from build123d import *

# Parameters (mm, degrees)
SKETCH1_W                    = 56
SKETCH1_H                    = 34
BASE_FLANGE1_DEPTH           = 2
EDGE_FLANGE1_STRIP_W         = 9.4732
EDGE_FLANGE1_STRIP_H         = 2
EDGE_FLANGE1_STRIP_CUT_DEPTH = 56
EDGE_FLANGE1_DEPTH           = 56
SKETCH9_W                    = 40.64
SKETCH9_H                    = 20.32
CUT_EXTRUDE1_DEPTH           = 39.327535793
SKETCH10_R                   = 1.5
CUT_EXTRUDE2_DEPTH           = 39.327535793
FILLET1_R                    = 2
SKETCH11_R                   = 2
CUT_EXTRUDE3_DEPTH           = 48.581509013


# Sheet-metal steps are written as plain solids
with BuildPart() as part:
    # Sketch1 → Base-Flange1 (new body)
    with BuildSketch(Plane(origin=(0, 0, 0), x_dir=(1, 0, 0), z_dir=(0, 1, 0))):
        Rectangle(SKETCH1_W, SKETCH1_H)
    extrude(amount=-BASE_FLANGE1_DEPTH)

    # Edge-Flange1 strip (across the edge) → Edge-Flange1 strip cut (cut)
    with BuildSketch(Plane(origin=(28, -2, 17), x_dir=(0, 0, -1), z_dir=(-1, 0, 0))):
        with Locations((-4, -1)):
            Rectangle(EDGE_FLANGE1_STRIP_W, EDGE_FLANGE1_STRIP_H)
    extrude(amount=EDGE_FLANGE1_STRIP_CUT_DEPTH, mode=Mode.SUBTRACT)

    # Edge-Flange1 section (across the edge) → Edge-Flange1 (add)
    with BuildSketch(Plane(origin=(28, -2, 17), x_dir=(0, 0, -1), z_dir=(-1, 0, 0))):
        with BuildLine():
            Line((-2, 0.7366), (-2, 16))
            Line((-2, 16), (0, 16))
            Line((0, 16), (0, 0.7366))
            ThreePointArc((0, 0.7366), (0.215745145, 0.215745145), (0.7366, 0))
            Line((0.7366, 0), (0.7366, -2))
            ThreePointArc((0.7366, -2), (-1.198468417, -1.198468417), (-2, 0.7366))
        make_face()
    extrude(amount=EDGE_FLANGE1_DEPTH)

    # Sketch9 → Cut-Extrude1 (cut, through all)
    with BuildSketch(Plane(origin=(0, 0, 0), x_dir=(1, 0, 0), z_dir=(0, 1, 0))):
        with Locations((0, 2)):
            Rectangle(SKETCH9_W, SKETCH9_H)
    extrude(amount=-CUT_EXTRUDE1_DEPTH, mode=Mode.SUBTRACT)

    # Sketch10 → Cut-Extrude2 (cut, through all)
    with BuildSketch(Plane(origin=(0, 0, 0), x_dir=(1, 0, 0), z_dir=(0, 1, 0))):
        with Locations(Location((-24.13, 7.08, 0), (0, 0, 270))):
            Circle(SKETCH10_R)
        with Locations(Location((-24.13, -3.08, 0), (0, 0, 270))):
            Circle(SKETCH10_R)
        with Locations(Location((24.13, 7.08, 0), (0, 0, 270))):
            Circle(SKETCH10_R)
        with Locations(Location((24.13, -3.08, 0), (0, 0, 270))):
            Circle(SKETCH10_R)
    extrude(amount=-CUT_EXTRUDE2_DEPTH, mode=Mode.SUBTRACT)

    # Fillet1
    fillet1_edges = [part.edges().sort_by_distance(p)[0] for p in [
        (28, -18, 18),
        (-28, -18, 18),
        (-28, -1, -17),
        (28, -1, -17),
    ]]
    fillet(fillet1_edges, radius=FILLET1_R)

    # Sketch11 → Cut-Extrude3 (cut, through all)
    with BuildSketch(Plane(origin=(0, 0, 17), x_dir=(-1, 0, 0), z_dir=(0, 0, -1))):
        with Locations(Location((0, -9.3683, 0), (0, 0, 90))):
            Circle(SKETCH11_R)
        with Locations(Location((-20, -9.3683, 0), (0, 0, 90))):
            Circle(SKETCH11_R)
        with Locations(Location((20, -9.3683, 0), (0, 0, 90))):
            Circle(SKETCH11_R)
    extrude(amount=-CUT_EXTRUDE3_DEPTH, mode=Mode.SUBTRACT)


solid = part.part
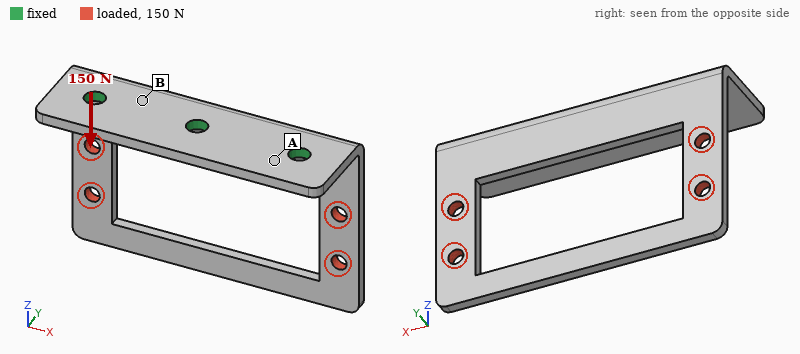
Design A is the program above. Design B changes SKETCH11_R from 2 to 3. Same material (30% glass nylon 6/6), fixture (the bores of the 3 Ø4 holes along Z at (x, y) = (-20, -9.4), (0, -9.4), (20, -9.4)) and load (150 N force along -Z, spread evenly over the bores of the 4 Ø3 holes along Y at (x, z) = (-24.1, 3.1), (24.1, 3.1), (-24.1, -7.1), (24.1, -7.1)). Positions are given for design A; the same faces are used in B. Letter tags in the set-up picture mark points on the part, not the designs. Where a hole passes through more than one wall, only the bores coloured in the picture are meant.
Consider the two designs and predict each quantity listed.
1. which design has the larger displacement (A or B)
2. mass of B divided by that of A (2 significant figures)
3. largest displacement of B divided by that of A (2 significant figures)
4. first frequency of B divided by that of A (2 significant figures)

A
0.98
0.74
1.0
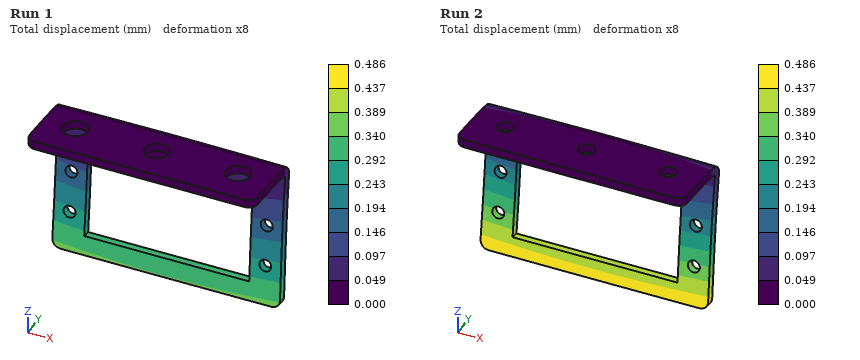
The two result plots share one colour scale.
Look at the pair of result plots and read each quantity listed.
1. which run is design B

Run 1
